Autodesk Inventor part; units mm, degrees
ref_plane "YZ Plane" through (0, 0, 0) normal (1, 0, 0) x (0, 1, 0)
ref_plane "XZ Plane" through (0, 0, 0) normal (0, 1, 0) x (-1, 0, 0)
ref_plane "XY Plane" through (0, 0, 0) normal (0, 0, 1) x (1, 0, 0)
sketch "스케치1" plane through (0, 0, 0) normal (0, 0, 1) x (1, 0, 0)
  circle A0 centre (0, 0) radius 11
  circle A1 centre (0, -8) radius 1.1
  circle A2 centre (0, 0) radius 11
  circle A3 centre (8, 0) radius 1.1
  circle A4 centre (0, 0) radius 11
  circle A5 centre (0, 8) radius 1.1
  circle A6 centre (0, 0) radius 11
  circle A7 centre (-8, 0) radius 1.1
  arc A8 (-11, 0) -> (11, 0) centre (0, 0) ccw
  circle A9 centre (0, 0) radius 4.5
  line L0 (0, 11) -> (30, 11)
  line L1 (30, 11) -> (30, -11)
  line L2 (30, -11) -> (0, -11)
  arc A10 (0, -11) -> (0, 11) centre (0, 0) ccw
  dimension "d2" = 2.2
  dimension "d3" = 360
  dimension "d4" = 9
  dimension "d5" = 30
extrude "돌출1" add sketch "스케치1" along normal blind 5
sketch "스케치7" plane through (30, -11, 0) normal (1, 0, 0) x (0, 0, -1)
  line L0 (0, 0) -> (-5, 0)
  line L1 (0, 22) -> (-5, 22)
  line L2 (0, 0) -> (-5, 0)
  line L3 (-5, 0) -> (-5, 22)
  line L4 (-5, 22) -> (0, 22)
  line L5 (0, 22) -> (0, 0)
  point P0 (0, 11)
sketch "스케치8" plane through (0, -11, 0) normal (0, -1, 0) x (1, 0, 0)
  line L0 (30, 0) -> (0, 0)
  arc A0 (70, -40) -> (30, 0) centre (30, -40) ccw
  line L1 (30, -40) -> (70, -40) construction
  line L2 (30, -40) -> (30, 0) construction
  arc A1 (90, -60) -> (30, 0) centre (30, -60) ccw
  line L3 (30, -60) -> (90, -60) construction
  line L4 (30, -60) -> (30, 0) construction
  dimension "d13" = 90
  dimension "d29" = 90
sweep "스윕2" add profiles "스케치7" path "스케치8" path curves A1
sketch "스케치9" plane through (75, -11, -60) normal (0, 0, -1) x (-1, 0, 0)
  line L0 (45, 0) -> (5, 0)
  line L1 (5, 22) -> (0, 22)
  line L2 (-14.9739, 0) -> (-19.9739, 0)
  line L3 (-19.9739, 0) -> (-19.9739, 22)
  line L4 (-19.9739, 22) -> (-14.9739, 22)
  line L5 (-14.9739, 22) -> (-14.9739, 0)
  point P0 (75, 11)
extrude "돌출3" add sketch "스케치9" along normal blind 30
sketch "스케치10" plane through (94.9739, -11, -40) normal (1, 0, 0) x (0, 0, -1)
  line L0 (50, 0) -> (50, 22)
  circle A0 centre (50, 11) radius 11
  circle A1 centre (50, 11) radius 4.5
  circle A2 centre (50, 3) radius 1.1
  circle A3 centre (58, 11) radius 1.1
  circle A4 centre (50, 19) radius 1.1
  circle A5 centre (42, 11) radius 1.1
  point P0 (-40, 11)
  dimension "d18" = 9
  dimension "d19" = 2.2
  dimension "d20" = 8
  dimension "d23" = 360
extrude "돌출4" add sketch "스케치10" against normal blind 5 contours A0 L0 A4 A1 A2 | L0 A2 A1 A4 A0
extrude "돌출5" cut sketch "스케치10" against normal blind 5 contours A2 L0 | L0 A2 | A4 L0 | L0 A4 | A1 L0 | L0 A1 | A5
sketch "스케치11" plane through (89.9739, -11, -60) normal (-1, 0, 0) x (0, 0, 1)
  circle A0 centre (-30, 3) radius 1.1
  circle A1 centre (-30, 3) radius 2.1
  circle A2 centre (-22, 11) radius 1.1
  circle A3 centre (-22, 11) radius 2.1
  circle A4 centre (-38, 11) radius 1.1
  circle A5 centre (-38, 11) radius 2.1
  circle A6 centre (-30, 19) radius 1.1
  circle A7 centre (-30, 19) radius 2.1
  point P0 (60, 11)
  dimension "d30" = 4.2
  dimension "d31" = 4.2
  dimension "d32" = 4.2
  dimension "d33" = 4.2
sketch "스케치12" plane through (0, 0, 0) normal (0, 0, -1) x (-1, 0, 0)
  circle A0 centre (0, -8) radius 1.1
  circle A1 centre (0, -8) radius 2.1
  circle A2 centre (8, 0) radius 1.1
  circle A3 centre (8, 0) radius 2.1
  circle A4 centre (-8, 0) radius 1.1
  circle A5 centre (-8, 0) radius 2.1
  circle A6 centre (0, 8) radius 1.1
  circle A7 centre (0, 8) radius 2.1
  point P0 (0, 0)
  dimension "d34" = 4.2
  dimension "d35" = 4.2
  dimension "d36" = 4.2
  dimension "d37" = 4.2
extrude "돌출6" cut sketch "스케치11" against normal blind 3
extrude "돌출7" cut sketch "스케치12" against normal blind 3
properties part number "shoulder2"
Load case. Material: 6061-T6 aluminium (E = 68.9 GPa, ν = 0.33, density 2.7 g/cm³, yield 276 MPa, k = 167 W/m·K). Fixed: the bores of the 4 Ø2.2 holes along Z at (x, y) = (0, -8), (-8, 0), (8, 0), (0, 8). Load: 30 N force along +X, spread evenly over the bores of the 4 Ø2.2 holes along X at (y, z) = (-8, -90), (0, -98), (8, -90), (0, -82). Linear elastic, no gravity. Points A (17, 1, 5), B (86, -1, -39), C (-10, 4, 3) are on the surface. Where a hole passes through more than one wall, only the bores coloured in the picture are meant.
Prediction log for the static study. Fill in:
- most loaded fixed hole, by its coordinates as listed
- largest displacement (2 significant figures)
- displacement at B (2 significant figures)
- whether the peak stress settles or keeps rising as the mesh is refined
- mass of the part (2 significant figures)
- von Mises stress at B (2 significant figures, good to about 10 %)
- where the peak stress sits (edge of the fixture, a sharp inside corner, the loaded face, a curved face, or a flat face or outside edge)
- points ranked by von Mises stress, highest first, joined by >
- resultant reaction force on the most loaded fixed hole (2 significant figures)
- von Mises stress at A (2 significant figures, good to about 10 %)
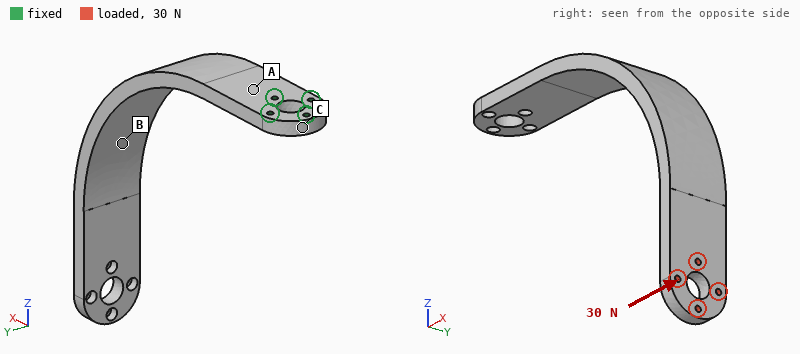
(8, 0)
1.8 mm
0.79 mm
keeps rising
49 g
18 MPa
edge of the fixture
A > B > C
340 N
28 MPa
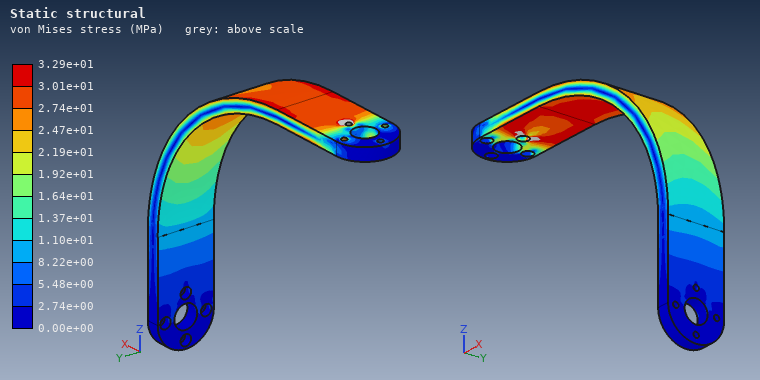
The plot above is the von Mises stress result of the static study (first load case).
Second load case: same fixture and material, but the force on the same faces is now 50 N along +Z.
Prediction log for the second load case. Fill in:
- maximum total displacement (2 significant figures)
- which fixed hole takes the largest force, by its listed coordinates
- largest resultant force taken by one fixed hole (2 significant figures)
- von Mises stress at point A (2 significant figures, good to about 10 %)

1.6 mm
(8, 0)
570 N
39 MPa
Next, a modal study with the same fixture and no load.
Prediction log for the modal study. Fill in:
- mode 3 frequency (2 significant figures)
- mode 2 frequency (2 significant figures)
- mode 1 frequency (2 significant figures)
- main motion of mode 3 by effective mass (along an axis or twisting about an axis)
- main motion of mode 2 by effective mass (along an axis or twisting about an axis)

690 Hz
310 Hz
180 Hz
along Z
along Y
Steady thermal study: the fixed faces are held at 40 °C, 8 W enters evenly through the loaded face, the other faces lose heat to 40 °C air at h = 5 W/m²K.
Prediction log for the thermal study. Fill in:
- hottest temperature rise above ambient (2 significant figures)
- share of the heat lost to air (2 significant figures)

64 K
18 %
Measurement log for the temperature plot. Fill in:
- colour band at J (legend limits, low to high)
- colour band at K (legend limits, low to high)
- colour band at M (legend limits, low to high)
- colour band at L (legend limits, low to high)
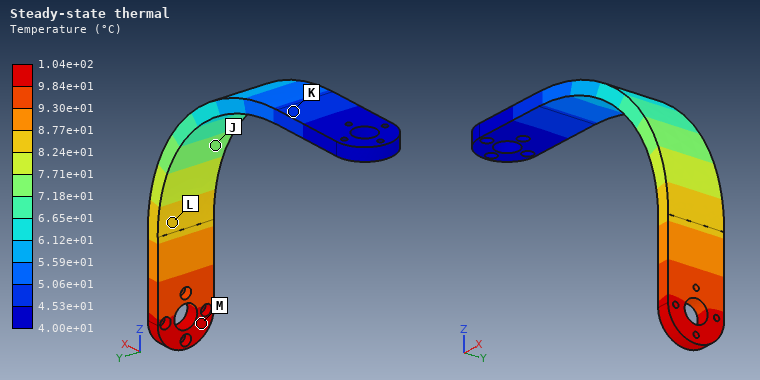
7.18e+01 to 7.71e+01 °C
4.53e+01 to 5.06e+01 °C
9.84e+01 to 1.04e+02 °C
8.24e+01 to 8.77e+01 °C
